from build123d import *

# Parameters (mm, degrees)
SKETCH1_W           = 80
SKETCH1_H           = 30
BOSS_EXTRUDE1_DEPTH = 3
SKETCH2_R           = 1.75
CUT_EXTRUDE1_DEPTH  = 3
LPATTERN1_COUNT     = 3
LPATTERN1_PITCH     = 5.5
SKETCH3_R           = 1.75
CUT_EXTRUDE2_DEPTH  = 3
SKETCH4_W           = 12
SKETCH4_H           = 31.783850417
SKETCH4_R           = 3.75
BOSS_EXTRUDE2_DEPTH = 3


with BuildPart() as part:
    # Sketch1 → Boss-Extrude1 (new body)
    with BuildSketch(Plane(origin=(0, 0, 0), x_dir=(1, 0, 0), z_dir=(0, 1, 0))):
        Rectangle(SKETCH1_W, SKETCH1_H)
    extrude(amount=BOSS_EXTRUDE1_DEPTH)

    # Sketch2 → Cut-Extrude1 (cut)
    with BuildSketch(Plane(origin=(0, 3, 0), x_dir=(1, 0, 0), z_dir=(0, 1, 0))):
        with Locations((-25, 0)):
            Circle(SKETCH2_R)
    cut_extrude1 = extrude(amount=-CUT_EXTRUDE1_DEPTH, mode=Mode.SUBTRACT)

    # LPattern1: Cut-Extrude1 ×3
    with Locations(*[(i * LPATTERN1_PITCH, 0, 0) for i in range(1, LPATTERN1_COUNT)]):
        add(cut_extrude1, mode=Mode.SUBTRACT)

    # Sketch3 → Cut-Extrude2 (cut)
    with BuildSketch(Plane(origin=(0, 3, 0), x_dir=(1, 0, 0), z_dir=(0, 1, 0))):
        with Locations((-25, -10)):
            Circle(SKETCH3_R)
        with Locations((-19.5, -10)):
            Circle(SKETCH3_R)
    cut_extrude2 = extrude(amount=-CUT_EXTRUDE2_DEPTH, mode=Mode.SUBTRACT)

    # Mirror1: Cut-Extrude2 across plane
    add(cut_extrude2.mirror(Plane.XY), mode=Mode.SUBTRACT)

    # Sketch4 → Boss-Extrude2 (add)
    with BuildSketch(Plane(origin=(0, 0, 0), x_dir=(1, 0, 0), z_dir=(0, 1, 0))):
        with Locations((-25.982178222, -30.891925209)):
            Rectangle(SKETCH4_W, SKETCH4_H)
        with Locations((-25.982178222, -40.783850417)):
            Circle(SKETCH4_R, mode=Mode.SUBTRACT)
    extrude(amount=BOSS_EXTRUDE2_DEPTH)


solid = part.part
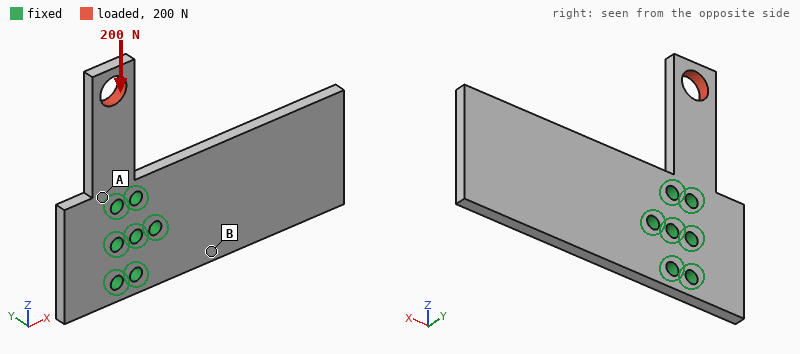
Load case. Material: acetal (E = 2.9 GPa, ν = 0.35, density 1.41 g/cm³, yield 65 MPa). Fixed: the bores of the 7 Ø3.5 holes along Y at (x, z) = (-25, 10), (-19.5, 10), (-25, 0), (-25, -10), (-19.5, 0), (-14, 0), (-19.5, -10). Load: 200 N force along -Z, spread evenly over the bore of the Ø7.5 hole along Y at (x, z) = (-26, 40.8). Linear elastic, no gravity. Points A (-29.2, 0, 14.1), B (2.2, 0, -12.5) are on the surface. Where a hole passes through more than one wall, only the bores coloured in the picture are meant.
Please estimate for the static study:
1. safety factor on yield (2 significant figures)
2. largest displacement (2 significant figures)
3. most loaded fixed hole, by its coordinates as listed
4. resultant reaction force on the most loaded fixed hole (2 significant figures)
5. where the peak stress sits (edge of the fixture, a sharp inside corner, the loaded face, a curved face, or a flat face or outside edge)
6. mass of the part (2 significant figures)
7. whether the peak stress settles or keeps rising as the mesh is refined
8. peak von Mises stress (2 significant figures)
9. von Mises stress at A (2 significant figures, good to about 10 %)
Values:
3.1
0.11 mm
(-25, 10)
140 N
the loaded face
11 g
settles
21 MPa
4.1 MPa
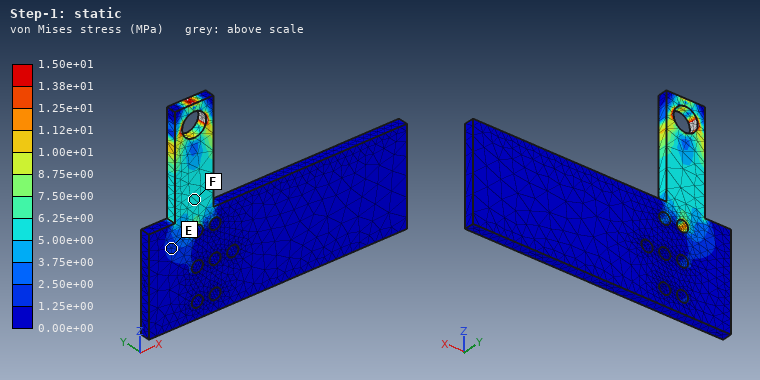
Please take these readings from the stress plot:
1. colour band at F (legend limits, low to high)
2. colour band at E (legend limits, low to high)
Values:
5.00e+00 to 6.25e+00 MPa
1.25e+00 to 2.50e+00 MPa
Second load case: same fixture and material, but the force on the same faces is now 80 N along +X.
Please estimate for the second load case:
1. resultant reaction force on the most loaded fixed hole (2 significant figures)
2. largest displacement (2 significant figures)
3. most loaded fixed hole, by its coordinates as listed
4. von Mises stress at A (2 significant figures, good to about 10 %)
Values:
200 N
0.87 mm
(-19.5, 10)
11 MPa
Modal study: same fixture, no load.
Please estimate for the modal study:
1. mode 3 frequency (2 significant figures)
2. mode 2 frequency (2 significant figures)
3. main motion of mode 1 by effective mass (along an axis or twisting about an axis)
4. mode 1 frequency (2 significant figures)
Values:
830 Hz
650 Hz
along Y
240 Hz
